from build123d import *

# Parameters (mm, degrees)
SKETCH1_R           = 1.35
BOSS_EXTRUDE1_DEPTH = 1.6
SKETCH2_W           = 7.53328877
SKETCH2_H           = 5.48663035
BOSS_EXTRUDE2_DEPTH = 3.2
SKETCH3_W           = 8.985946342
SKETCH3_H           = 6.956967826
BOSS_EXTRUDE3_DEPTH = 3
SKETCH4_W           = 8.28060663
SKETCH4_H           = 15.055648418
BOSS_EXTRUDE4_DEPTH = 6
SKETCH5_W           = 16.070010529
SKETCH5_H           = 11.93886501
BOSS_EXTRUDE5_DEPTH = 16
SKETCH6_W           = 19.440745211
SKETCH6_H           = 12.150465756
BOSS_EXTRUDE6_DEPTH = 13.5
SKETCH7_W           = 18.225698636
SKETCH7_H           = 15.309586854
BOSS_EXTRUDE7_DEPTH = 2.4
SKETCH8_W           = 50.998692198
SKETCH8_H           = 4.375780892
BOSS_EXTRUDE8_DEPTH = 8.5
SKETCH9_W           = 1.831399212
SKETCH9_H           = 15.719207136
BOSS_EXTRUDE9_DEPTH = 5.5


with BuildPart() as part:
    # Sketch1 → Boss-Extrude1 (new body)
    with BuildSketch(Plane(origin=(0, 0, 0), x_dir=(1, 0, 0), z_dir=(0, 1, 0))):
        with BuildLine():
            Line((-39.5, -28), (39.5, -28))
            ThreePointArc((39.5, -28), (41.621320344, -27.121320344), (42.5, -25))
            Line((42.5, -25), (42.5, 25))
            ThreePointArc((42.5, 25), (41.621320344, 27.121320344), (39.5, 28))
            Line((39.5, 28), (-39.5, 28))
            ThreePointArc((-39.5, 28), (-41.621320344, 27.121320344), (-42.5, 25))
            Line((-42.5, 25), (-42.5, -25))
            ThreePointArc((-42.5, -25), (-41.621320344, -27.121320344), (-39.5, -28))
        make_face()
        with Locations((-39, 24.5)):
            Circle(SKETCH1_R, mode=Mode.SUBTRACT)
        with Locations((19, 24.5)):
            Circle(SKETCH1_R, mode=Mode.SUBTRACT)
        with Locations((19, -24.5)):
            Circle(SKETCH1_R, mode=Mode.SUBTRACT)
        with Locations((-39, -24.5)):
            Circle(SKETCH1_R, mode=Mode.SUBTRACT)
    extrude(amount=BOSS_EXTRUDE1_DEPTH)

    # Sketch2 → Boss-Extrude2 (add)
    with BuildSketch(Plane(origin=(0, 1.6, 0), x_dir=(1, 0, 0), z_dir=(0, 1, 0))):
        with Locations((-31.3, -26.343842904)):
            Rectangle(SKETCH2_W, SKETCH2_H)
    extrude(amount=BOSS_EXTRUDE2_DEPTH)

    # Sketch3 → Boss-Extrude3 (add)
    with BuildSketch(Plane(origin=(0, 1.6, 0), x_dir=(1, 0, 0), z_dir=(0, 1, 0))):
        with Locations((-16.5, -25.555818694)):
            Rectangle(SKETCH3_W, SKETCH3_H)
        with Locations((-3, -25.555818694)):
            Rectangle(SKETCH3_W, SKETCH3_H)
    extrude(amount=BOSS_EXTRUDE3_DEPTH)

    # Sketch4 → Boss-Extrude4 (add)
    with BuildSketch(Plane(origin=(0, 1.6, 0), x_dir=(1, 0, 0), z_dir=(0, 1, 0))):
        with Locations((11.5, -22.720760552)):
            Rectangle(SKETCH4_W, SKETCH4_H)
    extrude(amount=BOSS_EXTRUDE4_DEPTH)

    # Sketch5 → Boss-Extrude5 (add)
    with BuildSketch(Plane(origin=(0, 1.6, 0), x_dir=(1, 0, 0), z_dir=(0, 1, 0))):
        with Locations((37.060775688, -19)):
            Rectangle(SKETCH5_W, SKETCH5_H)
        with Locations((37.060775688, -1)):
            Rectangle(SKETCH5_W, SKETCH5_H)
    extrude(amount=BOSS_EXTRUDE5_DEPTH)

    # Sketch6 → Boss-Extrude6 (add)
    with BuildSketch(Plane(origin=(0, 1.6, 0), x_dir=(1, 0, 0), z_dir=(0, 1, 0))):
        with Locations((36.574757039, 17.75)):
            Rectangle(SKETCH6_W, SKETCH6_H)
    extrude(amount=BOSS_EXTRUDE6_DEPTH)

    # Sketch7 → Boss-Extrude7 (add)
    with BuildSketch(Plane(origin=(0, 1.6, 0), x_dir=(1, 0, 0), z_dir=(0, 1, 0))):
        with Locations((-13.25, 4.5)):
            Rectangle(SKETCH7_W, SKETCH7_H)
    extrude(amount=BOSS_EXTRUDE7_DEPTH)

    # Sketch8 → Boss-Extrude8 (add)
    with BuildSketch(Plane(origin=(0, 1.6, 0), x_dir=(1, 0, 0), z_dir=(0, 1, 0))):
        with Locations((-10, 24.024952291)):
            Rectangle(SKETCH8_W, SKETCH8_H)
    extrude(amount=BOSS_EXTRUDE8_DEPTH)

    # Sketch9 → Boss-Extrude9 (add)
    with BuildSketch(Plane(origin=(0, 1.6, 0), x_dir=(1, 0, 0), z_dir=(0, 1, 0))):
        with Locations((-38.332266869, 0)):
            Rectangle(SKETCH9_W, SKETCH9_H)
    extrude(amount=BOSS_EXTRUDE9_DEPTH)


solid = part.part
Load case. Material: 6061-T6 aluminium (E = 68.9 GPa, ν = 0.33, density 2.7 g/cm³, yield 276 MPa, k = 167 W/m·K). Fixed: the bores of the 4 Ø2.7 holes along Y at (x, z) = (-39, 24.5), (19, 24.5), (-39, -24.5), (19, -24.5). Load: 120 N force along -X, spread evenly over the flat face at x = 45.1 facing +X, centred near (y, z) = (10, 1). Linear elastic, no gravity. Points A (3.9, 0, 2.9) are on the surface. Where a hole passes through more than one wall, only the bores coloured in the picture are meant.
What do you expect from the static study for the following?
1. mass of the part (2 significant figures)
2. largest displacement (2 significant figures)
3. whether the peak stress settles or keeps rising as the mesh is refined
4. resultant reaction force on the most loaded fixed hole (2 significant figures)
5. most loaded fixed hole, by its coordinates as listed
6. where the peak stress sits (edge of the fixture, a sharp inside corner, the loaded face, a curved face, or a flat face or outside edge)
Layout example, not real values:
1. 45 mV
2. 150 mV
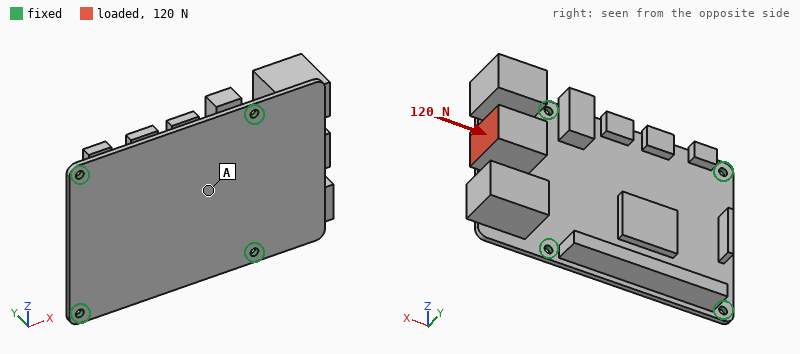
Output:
1. 56 g
2. 0.29 mm
3. keeps rising
4. 49 N
5. (19, 24.5)
6. edge of the fixture
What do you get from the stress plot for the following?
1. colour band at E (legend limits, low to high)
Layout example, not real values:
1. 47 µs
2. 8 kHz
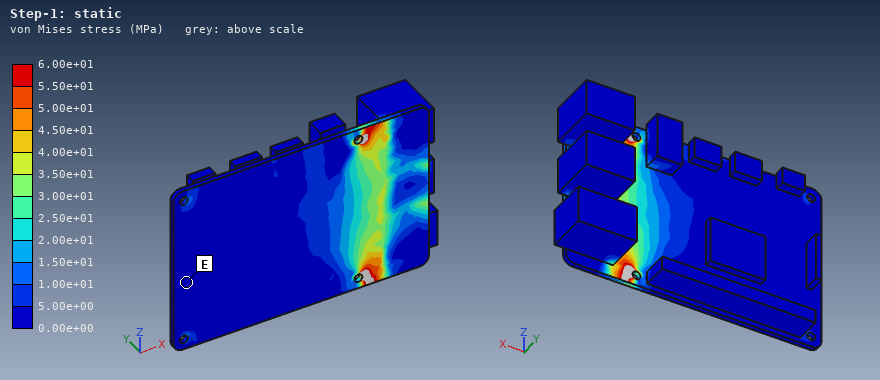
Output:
1. 0.00e+00 to 5.00e+00 MPa
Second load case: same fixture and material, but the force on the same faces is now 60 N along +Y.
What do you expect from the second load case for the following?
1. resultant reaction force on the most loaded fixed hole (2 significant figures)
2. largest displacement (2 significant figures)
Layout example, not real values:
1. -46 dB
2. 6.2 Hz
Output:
1. 40 N
2. 0.41 mm
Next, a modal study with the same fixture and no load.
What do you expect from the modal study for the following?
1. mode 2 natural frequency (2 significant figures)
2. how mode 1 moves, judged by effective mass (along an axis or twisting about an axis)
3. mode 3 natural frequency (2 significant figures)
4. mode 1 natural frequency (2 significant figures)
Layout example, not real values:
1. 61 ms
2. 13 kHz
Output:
1. 1600 Hz
2. along Y
3. 1800 Hz
4. 550 Hz
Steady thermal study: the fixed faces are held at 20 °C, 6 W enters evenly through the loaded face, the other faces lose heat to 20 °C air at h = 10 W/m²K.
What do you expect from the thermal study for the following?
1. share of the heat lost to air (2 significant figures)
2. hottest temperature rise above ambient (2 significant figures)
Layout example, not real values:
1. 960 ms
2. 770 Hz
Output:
1. 9.0 %
2. 14 K
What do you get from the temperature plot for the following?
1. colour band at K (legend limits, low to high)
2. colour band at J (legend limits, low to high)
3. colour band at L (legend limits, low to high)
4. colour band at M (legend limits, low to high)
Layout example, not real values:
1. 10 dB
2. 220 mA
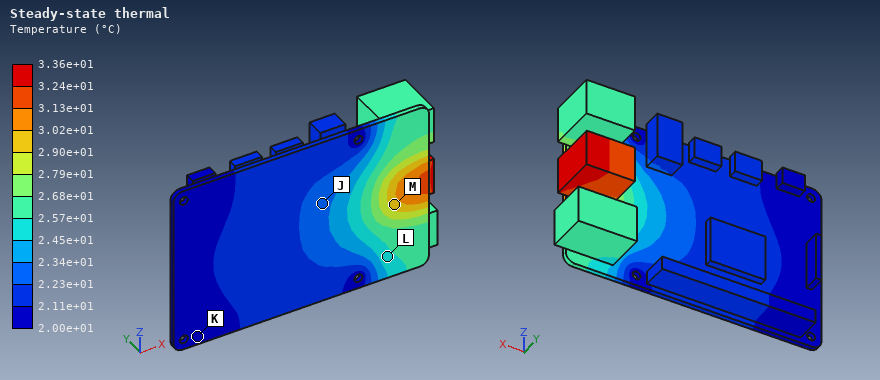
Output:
1. 2.00e+01 to 2.11e+01 °C
2. 2.23e+01 to 2.34e+01 °C
3. 2.45e+01 to 2.57e+01 °C
4. 2.90e+01 to 3.02e+01 °C
